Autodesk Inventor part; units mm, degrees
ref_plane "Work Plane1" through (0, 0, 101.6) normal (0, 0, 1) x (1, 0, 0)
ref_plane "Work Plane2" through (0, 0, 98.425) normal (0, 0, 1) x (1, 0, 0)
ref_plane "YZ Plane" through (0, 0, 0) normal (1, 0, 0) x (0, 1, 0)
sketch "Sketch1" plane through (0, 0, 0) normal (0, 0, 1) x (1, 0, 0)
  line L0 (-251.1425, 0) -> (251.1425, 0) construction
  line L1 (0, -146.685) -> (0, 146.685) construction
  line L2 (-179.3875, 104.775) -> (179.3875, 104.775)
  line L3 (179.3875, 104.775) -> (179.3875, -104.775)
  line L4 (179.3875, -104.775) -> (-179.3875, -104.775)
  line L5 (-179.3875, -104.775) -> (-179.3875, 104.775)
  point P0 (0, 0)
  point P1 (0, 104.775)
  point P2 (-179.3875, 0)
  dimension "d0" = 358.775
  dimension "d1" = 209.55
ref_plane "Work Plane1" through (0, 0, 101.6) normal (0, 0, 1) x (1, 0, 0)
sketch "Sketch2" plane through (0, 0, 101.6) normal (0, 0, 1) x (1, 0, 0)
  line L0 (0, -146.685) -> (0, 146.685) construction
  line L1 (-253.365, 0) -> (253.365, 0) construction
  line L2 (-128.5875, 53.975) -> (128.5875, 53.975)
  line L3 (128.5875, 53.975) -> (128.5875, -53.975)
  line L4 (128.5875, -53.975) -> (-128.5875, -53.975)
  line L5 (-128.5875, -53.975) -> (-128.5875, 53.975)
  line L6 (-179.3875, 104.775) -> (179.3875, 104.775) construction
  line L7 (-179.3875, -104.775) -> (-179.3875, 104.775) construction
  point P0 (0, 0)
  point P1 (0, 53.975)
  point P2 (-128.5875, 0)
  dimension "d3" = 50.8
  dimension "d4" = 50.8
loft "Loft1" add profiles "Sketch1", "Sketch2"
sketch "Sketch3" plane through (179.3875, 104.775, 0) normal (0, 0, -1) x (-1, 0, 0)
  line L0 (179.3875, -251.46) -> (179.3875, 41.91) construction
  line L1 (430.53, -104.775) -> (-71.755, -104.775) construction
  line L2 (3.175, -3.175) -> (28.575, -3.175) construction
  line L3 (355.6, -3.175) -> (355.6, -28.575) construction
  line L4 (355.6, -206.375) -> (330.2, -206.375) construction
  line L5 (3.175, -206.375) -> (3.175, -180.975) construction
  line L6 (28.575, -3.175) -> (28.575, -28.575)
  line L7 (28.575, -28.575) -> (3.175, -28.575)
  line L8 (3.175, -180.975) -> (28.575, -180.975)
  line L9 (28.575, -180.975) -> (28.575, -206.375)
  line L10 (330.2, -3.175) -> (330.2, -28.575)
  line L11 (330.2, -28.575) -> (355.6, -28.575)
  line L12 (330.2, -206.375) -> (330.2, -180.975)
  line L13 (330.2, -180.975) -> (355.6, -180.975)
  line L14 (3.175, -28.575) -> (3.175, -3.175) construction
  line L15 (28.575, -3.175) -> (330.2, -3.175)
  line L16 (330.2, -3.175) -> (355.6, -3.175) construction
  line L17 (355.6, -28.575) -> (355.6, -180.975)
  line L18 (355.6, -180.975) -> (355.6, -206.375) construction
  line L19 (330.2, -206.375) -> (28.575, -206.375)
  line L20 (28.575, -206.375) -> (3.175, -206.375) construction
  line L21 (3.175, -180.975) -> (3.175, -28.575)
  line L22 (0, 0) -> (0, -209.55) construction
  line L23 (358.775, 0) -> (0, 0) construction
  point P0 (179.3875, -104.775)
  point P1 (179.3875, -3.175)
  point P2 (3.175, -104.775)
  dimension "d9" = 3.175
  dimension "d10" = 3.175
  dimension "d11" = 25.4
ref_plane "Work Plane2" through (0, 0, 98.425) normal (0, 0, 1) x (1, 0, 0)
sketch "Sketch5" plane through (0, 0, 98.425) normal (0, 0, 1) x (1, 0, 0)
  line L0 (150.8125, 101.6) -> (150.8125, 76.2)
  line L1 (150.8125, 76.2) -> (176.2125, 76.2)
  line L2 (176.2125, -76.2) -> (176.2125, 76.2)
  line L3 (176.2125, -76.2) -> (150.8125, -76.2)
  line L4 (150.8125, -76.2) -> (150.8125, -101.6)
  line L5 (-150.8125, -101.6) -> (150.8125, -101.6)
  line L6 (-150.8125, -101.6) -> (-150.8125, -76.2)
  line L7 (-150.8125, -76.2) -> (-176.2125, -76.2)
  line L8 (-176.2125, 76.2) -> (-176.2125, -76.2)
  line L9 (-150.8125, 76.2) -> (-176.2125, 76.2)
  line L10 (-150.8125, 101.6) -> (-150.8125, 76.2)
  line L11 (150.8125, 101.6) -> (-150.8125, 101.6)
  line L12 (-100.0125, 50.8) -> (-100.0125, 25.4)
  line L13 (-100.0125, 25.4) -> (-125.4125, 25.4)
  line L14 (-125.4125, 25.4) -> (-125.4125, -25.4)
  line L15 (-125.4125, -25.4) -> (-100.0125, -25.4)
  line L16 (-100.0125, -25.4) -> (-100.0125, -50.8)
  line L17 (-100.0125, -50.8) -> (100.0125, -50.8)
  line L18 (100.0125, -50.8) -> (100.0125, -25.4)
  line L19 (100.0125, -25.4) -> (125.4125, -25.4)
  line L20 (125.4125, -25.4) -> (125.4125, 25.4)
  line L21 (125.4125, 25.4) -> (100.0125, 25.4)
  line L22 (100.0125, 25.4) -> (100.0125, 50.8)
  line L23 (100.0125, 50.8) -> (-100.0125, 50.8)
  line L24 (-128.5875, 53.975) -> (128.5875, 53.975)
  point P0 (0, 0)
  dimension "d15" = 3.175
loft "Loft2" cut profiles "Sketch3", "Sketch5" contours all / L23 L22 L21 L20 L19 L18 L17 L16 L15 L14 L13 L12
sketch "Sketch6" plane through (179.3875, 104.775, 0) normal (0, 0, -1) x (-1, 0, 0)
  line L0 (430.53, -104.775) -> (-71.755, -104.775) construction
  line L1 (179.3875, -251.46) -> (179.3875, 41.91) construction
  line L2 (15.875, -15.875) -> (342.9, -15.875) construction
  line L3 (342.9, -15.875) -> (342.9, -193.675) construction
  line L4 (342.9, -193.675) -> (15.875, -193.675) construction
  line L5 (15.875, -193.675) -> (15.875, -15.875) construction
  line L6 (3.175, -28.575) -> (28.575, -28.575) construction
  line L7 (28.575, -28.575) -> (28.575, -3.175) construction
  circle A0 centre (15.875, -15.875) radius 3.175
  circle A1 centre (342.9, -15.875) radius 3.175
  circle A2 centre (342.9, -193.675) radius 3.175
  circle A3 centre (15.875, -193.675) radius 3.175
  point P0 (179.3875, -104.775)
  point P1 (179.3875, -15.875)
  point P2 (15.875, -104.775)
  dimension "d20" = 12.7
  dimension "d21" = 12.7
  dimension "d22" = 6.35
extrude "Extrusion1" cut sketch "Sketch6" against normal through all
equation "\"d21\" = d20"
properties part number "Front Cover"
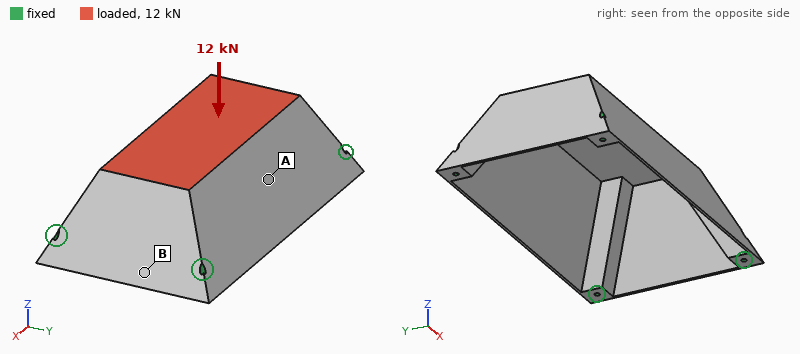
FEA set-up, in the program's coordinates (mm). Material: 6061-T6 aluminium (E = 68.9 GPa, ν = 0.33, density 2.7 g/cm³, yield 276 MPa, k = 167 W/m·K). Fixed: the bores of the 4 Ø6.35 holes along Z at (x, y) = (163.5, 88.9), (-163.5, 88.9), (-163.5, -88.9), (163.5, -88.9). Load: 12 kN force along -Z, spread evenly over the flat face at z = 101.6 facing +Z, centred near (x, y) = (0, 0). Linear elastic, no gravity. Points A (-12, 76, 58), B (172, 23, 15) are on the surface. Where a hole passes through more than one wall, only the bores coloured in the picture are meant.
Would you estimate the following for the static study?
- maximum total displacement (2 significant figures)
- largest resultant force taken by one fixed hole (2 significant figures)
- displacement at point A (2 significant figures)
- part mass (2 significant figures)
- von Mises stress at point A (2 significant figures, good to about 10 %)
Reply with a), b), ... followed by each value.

a) 1.2 mm
b) 4.3 kN
c) 0.73 mm
d) 1.9 kg
e) 29 MPa
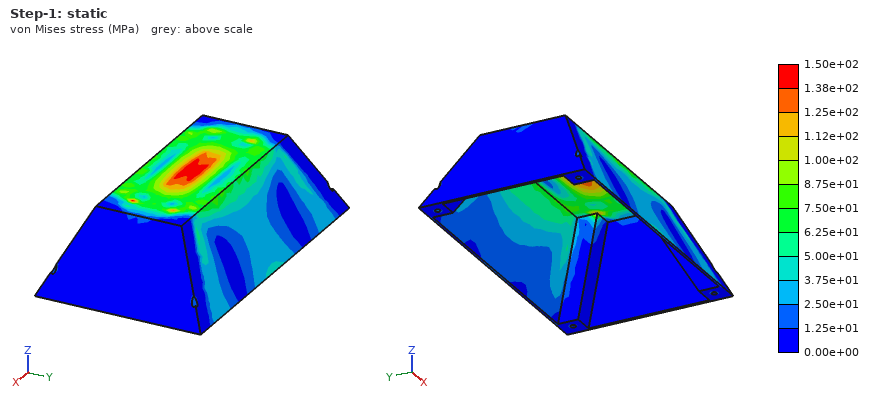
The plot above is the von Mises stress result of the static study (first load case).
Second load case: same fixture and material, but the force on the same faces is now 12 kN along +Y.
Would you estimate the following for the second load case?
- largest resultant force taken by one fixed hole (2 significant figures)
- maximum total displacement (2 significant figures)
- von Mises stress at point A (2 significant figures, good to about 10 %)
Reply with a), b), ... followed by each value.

a) 4.2 kN
b) 0.12 mm
c) 7.7 MPa
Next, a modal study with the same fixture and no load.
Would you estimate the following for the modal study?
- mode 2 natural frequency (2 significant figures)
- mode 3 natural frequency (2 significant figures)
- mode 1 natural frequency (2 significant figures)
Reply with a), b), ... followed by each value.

a) 390 Hz
b) 790 Hz
c) 370 Hz
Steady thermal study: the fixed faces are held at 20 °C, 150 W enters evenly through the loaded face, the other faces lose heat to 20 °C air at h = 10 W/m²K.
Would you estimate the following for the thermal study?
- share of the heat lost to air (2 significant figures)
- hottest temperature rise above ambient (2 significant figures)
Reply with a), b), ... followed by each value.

a) 25 %
b) 43 K
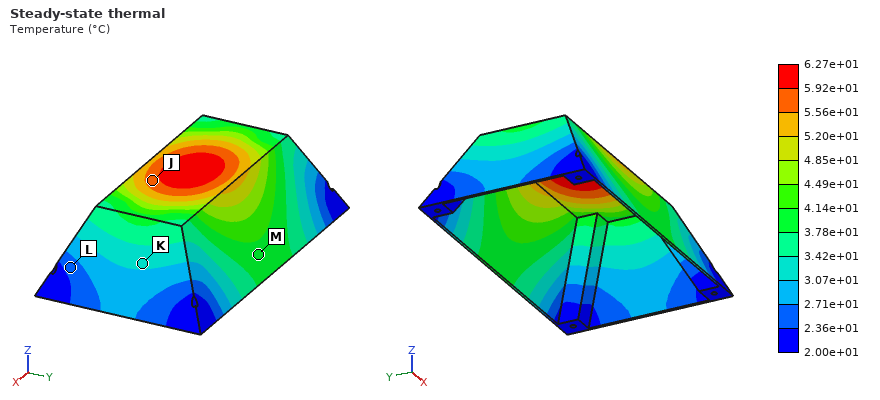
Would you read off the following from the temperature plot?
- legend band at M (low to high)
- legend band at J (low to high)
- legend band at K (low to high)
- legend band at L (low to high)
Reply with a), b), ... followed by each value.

a) 3.78e+01 to 4.14e+01 °C
b) 5.56e+01 to 5.92e+01 °C
c) 3.07e+01 to 3.42e+01 °C
d) 2.36e+01 to 2.71e+01 °C
